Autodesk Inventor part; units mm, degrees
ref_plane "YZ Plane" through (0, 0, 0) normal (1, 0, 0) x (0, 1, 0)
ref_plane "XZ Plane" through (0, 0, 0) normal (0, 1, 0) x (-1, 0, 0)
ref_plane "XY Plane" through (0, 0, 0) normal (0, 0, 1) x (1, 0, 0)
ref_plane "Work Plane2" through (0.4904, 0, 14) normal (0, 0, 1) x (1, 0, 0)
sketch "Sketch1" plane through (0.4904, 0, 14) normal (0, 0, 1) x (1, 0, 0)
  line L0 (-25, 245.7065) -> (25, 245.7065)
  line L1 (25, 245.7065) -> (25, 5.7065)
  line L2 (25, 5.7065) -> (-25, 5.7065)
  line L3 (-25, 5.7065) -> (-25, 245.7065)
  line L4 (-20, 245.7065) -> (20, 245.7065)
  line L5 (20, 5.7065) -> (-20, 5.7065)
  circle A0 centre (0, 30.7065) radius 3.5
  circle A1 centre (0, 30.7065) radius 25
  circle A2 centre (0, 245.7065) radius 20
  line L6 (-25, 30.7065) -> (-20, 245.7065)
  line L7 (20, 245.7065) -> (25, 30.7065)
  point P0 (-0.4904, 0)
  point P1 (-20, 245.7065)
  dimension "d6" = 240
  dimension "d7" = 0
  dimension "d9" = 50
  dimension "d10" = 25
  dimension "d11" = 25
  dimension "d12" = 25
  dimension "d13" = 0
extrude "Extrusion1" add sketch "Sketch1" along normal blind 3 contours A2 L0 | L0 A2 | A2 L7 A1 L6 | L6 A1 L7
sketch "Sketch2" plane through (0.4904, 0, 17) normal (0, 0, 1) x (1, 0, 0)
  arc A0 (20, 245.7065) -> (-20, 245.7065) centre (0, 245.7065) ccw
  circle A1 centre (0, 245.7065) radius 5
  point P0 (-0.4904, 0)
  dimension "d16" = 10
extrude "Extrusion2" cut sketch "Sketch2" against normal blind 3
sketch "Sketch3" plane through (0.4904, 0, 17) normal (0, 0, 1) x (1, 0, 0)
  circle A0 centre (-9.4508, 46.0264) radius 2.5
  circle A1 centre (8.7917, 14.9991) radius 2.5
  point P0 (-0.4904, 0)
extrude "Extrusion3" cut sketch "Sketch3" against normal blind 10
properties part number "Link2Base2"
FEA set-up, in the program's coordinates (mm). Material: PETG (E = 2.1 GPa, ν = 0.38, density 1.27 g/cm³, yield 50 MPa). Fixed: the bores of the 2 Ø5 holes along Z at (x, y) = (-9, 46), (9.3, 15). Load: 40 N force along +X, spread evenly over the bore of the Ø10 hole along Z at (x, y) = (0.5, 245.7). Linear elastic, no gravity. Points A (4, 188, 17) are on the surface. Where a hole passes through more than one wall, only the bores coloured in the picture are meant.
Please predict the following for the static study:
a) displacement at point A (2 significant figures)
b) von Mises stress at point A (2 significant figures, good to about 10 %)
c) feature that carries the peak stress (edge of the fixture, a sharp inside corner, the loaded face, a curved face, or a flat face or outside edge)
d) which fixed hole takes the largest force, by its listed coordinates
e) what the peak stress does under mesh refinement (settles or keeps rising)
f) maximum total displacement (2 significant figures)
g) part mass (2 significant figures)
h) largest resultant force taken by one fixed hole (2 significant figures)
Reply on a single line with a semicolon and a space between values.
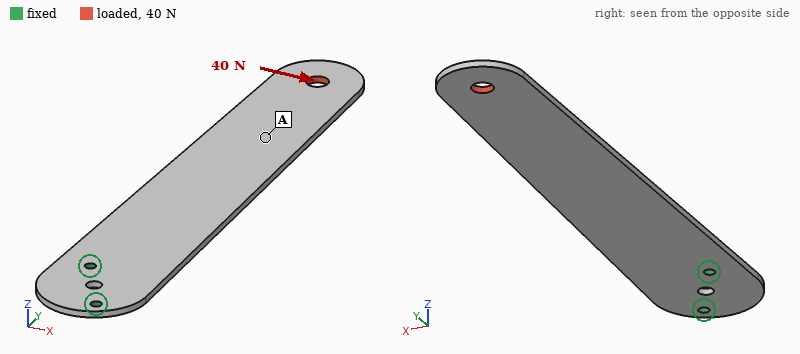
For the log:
1.6 mm; 0.85 MPa; edge of the fixture; (-9, 46); keeps rising; 3.0 mm; 42 g; 240 N
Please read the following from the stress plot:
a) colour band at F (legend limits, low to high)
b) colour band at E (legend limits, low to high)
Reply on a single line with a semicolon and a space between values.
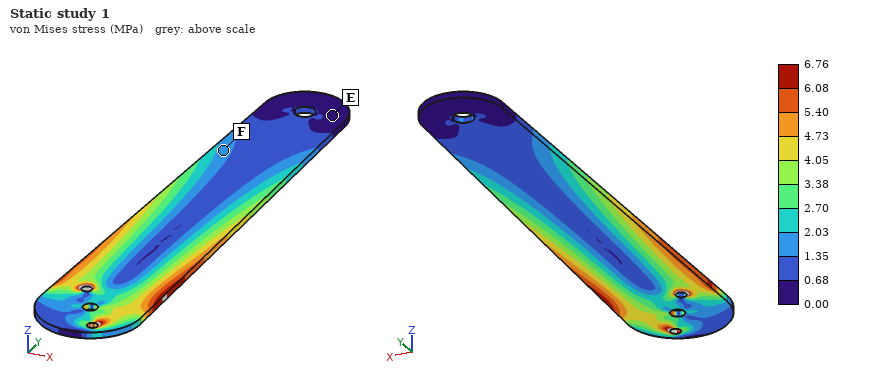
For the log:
1.35 to 2.03 MPa; 0.00 to 0.68 MPa
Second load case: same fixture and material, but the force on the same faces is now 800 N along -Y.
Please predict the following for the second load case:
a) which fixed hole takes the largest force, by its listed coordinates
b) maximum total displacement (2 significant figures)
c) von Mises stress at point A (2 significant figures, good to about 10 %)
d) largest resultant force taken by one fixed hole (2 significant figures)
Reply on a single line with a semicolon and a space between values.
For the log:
(-9, 46); 0.83 mm; 6.2 MPa; 520 N
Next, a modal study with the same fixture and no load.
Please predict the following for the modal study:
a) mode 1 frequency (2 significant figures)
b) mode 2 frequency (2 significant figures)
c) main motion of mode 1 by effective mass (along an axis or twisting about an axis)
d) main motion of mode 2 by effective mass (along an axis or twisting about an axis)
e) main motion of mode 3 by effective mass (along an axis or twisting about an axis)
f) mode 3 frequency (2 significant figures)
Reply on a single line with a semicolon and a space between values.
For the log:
15 Hz; 85 Hz; along Z; along Z; twisting about Y; 130 Hz
